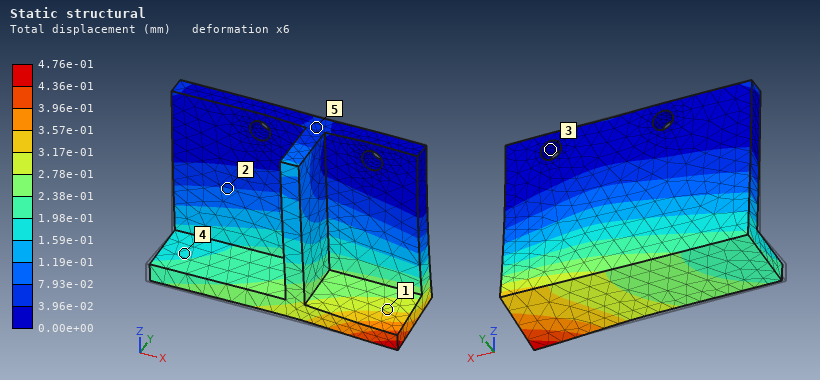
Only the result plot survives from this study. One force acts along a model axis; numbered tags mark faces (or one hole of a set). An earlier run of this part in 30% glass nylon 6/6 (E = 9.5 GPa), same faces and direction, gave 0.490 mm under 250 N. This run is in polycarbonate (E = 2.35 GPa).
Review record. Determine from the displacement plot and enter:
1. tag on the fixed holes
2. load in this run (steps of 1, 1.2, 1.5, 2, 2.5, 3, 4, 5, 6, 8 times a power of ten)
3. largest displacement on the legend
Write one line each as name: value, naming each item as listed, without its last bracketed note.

tag on the fixed holes: 3
load in this run: 60 N
largest displacement on the legend: 4.76e-01 mm
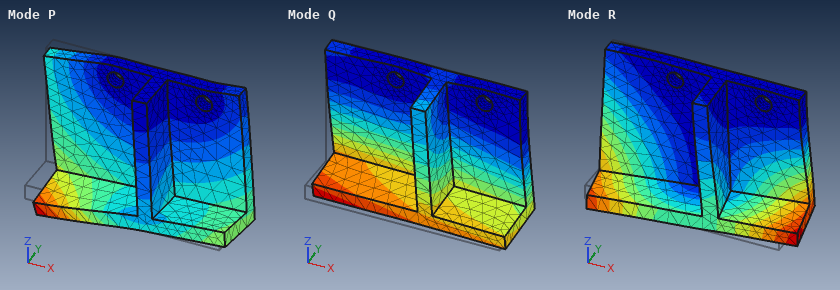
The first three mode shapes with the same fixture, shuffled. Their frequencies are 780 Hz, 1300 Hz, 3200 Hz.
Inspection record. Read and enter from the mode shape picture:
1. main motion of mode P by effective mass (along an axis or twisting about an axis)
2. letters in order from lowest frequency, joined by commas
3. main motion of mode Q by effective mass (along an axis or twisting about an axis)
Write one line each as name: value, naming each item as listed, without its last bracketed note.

main motion of mode P by effective mass: along X
letters in order from lowest frequency, joined by commas: Q, R, P
main motion of mode Q by effective mass: along Y
